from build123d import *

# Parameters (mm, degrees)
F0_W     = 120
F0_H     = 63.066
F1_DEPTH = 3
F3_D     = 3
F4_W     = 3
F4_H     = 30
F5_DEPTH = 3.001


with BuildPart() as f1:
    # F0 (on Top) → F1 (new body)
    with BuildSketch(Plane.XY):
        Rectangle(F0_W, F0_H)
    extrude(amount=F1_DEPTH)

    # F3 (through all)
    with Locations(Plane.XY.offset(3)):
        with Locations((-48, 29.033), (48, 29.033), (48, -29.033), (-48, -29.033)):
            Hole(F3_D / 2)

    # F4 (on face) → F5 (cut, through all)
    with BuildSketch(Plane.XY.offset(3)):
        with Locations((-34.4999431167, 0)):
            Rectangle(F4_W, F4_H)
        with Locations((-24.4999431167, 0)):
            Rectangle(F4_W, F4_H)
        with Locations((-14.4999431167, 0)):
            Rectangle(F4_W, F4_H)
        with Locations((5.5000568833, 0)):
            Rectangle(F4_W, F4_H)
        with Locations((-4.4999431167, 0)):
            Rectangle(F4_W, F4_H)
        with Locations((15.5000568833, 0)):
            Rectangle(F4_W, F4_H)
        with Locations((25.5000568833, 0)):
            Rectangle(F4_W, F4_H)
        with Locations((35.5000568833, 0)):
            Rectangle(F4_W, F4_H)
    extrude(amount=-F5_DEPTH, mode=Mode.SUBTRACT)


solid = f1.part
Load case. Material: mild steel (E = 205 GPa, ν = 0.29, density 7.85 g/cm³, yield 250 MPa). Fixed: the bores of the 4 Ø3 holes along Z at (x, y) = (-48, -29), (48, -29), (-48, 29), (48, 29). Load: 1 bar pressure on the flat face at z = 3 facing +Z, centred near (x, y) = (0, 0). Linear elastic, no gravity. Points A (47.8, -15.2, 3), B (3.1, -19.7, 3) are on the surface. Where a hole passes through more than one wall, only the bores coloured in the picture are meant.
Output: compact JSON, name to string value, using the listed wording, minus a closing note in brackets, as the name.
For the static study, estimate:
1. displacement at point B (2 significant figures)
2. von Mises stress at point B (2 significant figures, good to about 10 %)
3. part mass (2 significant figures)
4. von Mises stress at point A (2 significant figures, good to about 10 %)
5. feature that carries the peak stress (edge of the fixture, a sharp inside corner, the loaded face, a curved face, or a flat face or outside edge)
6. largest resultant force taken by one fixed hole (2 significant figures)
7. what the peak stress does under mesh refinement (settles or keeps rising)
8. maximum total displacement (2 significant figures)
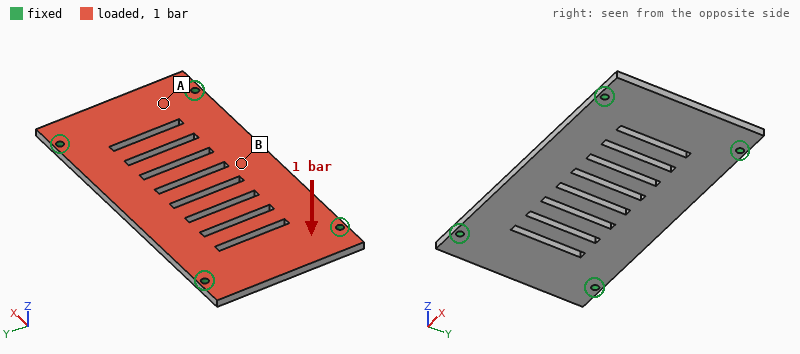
{"displacement at point B": "84 µm", "von Mises stress at point B": "38 MPa", "part mass": "160 g", "von Mises stress at point A": "21 MPa", "feature that carries the peak stress": "edge of the fixture", "largest resultant force taken by one fixed hole": "170 N", "what the peak stress does under mesh refinement": "keeps rising", "maximum total displacement": "94 µm"}
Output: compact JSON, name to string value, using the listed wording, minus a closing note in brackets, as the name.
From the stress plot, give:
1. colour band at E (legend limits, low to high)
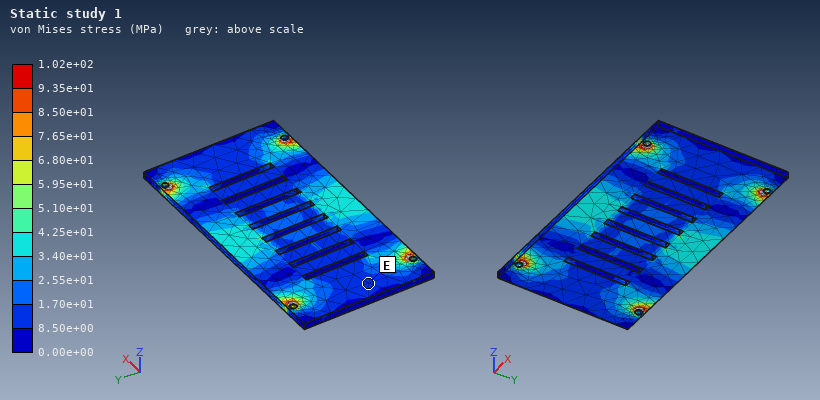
{"colour band at E": "8.50e+00 to 1.70e+01 MPa"}
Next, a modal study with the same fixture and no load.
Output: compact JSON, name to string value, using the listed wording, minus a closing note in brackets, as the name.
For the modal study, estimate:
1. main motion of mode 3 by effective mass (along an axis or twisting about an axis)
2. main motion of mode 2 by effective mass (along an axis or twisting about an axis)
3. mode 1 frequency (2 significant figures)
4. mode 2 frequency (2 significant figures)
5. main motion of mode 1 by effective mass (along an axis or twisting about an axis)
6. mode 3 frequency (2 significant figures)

{"main motion of mode 3 by effective mass": "twisting about Y", "main motion of mode 2 by effective mass": "twisting about X", "mode 1 frequency": "1300 Hz", "mode 2 frequency": "2200 Hz", "main motion of mode 1 by effective mass": "along Z", "mode 3 frequency": "3100 Hz"}
